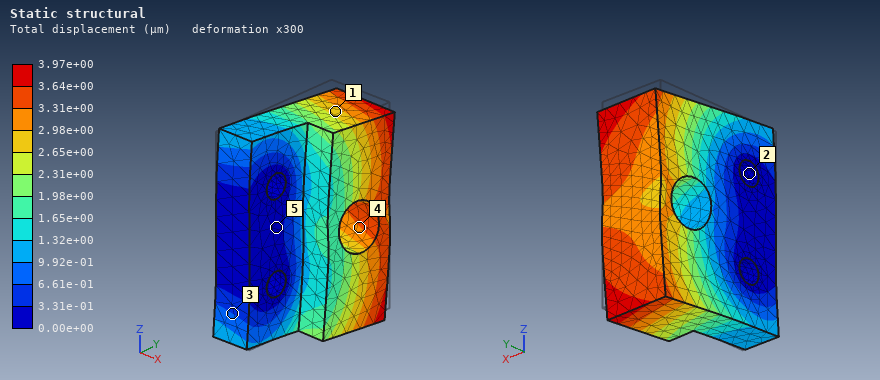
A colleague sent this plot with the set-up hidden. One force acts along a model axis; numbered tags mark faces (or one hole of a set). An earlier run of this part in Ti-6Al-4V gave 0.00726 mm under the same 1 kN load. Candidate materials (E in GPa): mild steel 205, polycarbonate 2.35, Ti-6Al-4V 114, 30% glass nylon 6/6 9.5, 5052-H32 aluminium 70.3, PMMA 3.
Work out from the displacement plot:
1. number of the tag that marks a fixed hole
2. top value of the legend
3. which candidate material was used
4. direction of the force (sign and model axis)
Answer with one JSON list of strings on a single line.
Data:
["2", "3.97e+00 µm", "mild steel", "-Z"]
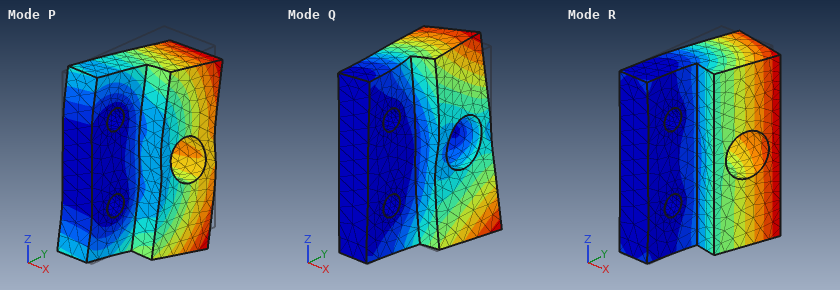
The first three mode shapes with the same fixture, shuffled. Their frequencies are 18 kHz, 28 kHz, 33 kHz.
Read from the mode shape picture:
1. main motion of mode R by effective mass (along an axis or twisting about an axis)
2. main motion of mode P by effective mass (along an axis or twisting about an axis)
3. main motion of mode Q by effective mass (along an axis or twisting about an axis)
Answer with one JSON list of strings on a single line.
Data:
["along X", "along Z", "twisting about Y"]
